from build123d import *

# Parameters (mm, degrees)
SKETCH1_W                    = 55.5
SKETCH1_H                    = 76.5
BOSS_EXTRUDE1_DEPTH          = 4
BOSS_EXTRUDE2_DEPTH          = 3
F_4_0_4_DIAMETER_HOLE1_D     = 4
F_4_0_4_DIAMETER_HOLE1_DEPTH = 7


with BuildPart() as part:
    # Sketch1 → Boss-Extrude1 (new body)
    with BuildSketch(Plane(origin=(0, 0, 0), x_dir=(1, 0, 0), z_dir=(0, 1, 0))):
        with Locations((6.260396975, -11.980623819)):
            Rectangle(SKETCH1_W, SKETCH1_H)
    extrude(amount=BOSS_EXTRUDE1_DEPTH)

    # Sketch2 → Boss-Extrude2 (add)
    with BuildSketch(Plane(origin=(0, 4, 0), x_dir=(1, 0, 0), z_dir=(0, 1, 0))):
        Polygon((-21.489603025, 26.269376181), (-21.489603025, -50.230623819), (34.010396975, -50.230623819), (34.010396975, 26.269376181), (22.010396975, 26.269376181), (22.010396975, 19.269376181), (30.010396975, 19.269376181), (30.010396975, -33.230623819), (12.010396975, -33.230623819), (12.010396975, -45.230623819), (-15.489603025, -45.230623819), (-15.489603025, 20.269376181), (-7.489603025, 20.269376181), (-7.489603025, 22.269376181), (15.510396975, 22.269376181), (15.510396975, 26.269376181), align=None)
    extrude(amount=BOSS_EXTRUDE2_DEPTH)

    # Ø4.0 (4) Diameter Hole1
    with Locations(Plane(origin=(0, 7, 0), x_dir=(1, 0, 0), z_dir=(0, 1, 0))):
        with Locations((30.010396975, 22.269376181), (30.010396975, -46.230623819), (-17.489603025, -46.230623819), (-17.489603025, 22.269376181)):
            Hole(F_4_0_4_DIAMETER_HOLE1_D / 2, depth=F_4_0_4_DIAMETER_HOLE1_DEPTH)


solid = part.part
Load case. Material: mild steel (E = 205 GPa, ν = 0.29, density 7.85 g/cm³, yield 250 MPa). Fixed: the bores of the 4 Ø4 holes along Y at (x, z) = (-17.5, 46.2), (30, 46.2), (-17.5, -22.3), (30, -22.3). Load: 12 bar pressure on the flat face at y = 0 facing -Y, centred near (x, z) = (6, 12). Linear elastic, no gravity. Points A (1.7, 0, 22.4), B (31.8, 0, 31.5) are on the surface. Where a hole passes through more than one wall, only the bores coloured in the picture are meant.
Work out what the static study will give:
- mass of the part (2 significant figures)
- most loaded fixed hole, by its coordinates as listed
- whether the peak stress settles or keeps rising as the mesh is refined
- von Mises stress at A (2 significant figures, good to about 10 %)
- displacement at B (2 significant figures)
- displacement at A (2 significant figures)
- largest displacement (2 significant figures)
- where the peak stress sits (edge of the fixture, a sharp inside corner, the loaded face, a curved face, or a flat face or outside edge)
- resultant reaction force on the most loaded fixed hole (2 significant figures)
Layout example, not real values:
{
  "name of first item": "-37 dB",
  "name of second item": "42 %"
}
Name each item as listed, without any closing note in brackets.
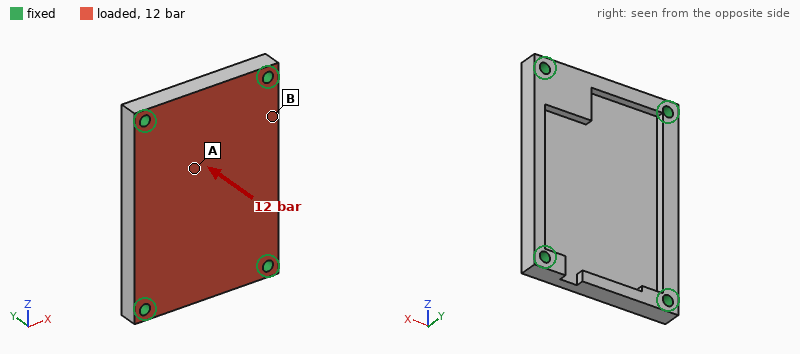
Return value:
{
  "mass of the part": "160 g",
  "most loaded fixed hole, by its coordinates as listed": "(30, 46.2)",
  "whether the peak stress settles or keeps rising as the mesh is refined": "keeps rising",
  "von Mises stress at A": "51 MPa",
  "displacement at B": "13 µm",
  "displacement at A": "42 µm",
  "largest displacement": "50 µm",
  "where the peak stress sits": "edge of the fixture",
  "resultant reaction force on the most loaded fixed hole": "1.6 kN"
}
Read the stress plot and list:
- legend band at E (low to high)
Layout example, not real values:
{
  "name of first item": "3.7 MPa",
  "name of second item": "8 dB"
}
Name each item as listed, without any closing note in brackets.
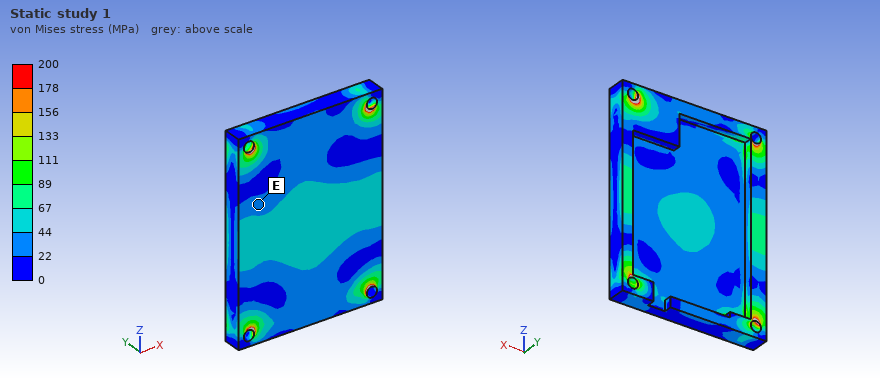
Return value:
{
  "legend band at E": "22 to 44 MPa"
}
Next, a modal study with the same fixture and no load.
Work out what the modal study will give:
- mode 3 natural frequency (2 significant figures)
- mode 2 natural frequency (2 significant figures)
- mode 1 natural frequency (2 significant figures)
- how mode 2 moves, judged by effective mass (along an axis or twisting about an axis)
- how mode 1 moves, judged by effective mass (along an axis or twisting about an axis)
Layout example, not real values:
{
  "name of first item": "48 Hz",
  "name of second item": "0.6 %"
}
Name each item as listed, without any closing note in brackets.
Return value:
{
  "mode 3 natural frequency": "11 kHz",
  "mode 2 natural frequency": "7800 Hz",
  "mode 1 natural frequency": "5200 Hz",
  "how mode 2 moves, judged by effective mass": "twisting about Z",
  "how mode 1 moves, judged by effective mass": "along Y"
}
